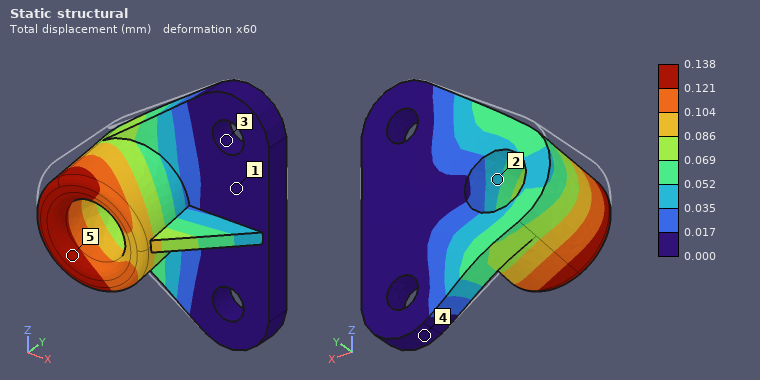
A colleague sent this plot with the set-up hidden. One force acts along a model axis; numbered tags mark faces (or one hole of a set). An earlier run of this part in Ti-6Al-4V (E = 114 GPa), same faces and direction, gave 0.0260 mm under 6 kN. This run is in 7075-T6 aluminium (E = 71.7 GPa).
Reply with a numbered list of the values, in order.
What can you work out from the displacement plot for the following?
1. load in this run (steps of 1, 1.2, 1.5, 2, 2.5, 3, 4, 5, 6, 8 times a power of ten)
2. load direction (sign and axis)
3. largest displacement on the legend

1. 20 kN
2. -Z
3. 0.138 mm
